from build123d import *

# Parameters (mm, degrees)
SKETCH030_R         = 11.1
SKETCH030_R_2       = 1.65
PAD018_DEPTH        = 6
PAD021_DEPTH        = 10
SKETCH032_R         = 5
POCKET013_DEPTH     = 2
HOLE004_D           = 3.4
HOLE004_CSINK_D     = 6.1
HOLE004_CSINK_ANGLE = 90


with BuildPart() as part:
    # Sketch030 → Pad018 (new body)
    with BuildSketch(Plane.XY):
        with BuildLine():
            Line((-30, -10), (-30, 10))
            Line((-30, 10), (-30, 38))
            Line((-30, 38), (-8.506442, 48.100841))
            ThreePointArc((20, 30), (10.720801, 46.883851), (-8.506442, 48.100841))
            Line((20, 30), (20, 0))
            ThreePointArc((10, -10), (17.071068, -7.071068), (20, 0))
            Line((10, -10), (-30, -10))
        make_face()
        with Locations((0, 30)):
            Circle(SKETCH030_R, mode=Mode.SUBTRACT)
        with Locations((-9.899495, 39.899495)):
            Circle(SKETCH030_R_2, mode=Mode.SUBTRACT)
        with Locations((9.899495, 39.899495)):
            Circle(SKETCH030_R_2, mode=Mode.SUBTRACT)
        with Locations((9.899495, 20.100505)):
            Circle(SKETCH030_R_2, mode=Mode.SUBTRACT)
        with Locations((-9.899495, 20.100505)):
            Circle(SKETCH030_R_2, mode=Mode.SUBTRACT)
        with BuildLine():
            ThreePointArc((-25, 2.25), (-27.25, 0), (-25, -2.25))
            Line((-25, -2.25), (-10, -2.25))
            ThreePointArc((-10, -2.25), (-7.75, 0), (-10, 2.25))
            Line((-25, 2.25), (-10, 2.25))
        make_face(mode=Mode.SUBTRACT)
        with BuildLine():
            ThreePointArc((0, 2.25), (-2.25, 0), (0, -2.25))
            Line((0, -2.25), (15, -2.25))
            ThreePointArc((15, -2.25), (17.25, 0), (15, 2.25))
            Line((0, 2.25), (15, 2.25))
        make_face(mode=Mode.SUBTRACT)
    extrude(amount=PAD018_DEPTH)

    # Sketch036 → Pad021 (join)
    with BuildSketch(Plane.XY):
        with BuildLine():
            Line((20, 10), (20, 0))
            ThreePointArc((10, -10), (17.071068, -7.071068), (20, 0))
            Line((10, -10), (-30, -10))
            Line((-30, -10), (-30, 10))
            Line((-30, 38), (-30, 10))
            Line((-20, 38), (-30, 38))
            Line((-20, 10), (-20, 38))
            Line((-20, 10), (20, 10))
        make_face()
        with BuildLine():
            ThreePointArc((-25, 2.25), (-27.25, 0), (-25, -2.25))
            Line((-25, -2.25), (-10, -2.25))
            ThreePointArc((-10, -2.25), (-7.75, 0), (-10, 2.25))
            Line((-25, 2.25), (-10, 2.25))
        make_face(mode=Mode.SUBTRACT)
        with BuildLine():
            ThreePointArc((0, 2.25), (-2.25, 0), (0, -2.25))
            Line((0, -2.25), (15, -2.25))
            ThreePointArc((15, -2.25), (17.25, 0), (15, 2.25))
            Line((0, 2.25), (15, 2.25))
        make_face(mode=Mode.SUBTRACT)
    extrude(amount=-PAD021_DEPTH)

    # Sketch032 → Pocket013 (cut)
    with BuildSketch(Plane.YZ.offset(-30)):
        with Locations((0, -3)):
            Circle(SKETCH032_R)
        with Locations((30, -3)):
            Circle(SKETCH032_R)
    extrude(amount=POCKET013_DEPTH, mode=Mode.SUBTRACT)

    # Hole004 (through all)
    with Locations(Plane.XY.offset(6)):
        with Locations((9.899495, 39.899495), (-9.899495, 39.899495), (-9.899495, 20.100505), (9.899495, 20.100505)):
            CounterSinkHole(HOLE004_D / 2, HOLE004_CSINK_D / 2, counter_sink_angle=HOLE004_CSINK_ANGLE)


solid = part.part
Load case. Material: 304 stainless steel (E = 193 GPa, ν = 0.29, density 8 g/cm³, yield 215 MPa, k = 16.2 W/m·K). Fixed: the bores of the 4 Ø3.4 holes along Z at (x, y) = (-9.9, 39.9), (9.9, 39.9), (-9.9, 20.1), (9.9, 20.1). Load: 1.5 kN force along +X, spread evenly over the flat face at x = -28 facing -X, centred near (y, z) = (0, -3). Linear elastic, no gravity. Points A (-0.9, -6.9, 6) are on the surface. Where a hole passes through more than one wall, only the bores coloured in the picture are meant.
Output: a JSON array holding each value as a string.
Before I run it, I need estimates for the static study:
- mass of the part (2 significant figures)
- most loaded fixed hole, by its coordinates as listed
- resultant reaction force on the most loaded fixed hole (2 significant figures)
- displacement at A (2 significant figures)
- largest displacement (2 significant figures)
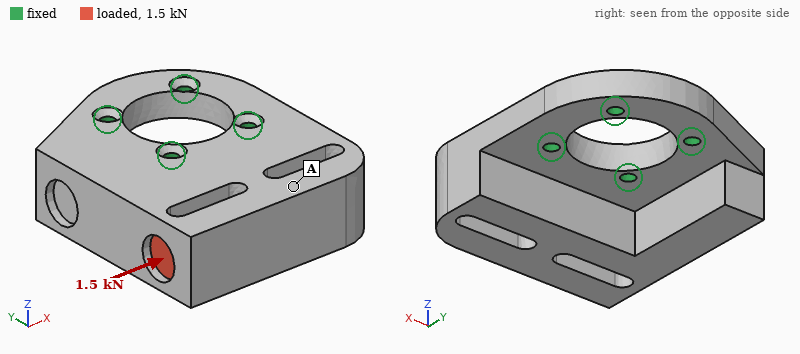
["190 g", "(-9.9, 20.1)", "1.4 kN", "3.3 µm", "9.6 µm"]
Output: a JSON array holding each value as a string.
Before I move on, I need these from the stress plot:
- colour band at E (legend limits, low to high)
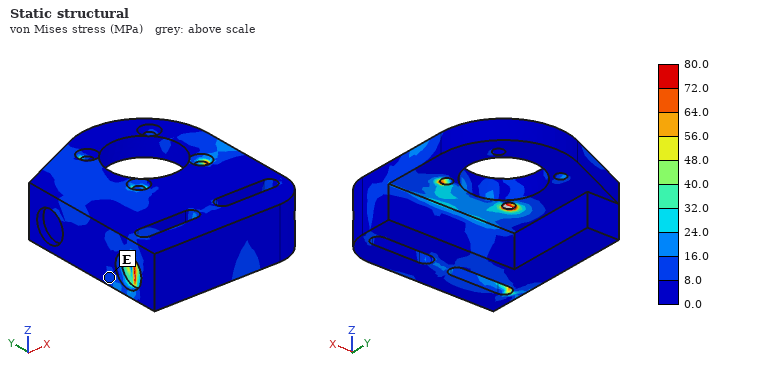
["8.0 to 16.0 MPa"]
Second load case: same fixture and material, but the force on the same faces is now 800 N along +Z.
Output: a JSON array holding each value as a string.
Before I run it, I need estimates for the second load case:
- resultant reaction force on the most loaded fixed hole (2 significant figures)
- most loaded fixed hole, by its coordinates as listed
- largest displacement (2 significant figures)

["1.6 kN", "(-9.9, 20.1)", "39 µm"]
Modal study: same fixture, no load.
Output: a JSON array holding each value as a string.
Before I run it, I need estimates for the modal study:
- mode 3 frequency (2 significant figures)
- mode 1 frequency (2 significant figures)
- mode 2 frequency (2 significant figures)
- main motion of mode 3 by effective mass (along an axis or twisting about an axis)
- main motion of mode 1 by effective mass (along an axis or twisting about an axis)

["9400 Hz", "3400 Hz", "5400 Hz", "along X", "along Z"]
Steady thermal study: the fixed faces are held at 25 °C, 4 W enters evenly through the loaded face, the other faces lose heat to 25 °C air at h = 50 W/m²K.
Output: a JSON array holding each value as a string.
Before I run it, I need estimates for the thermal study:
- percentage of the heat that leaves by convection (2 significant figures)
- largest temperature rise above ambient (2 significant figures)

["61 %", "31 K"]
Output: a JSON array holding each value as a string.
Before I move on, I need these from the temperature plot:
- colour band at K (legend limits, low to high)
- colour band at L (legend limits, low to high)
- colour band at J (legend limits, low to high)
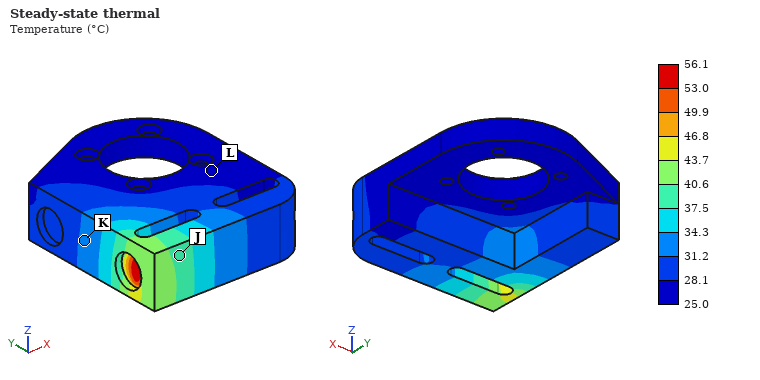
["31.2 to 34.3 °C", "25.0 to 28.1 °C", "37.5 to 40.6 °C"]
